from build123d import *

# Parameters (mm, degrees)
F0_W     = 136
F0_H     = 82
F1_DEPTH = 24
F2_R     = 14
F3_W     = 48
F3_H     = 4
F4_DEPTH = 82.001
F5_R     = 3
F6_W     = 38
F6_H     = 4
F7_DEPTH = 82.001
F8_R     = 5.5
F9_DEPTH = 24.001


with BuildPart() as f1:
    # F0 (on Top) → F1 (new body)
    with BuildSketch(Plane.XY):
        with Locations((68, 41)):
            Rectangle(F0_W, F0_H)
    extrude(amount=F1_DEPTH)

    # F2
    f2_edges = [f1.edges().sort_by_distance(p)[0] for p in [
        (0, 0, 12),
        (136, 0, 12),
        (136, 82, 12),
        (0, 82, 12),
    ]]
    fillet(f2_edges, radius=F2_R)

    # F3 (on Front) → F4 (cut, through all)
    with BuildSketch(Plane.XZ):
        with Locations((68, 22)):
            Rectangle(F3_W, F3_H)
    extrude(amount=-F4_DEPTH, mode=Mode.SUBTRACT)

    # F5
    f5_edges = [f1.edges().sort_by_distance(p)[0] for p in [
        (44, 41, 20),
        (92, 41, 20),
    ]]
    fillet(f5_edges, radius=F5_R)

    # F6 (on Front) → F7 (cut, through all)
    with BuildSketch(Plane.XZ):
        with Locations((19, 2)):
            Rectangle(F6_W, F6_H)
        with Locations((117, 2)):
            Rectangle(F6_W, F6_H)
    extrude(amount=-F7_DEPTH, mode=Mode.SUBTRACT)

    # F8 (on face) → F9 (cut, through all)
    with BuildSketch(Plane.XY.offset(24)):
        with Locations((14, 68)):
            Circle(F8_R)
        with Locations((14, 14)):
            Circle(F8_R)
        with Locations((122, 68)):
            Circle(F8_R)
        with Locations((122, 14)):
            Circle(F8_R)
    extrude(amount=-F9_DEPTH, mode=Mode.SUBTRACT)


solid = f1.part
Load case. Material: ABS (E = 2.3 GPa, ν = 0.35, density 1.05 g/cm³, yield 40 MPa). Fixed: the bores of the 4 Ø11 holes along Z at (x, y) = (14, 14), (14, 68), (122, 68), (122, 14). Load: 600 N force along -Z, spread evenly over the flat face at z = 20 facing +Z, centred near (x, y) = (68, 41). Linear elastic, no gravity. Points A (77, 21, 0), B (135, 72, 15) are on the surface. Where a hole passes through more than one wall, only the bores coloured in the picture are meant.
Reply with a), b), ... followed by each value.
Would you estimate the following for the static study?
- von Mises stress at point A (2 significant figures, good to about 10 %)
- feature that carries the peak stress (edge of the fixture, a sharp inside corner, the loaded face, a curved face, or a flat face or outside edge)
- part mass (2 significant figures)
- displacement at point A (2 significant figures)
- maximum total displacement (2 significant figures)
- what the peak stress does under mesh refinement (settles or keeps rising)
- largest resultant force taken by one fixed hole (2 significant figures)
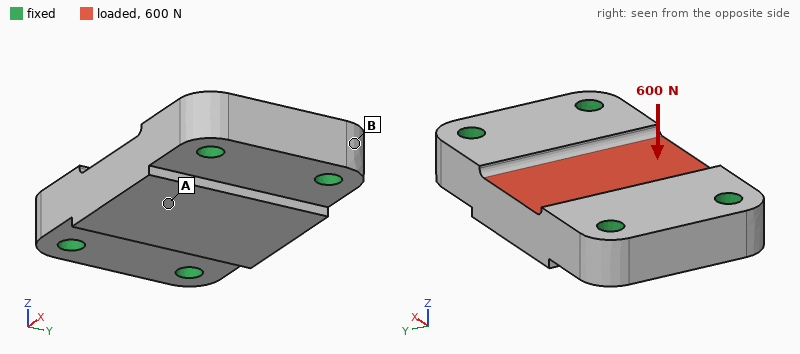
a) 0.90 MPa
b) edge of the fixture
c) 230 g
d) 33 µm
e) 39 µm
f) keeps rising
g) 170 N
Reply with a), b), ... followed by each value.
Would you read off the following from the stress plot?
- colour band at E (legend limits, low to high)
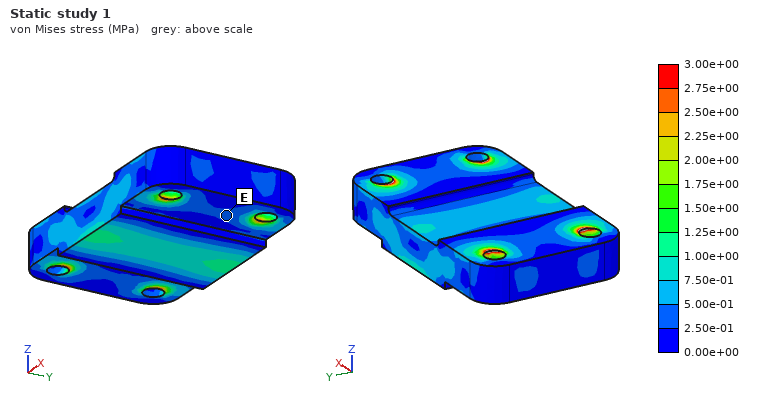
a) 2.50e-01 to 5.00e-01 MPa
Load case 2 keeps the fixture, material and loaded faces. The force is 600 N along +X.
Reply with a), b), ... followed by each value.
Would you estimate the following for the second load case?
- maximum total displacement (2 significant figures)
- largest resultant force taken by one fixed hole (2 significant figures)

a) 6.5 µm
b) 150 N
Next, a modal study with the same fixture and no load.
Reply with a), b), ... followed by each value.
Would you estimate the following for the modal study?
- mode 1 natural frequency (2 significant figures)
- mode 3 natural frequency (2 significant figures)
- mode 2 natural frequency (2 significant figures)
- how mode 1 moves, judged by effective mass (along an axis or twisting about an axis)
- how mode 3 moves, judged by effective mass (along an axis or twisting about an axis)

a) 2200 Hz
b) 3700 Hz
c) 2800 Hz
d) along Z
e) along Y
